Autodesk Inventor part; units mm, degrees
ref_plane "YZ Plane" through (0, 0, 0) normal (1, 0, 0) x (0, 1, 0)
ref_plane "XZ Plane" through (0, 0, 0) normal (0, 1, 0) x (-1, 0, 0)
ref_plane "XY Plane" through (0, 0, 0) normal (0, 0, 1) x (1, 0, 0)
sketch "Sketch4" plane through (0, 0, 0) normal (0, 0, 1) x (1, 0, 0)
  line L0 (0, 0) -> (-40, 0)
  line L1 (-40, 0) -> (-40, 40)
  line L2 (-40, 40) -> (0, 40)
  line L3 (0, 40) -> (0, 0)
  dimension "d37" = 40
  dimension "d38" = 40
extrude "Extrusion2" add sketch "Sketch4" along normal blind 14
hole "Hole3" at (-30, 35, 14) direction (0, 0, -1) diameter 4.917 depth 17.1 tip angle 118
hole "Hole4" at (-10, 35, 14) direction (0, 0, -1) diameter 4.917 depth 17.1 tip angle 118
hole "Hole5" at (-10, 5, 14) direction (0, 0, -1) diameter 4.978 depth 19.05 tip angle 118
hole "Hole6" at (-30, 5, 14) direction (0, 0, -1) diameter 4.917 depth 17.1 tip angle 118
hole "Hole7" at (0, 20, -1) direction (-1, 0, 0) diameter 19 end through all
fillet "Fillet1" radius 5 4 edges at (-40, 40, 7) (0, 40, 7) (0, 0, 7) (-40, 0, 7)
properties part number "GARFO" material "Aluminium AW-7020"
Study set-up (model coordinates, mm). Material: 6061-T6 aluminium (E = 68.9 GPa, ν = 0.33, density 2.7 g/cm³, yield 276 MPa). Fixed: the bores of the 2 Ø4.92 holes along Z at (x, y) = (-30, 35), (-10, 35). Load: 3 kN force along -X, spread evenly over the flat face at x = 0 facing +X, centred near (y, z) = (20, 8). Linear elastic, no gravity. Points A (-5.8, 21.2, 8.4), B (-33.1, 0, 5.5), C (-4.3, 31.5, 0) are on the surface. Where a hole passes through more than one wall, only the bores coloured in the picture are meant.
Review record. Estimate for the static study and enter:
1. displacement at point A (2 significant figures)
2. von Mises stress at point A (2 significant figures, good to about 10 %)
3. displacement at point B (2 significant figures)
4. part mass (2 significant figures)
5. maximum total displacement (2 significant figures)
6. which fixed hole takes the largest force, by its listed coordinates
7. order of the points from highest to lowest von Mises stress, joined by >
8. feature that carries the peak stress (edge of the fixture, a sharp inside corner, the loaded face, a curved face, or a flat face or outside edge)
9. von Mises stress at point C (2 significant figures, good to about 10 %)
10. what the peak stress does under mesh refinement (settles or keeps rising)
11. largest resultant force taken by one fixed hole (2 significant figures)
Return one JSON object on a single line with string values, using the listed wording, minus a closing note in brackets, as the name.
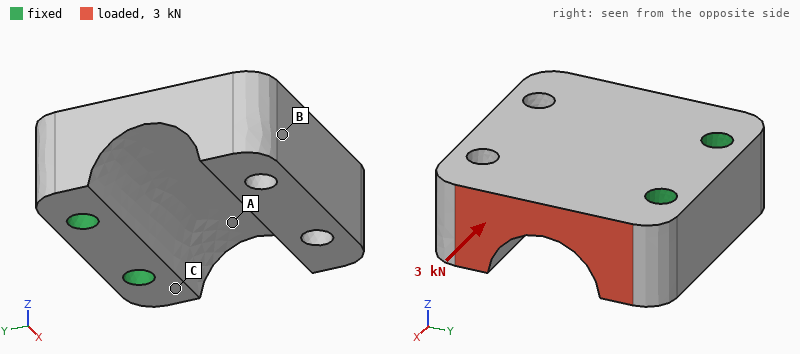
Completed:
{"displacement at point A": "9.0 µm", "von Mises stress at point A": "22 MPa", "displacement at point B": "18 µm", "part mass": "44 g", "maximum total displacement": "22 µm", "which fixed hole takes the largest force, by its listed coordinates": "(-10, 35)", "order of the points from highest to lowest von Mises stress, joined by >": "A > C > B", "feature that carries the peak stress": "edge of the fixture", "von Mises stress at point C": "12 MPa", "what the peak stress does under mesh refinement": "keeps rising", "largest resultant force taken by one fixed hole": "2.6 kN"}
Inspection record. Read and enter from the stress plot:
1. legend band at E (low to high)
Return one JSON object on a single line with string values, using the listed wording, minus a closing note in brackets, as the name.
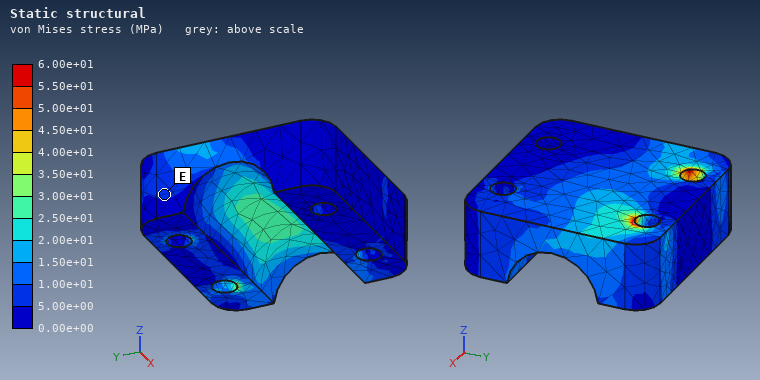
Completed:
{"legend band at E": "5.00e+00 to 1.00e+01 MPa"}
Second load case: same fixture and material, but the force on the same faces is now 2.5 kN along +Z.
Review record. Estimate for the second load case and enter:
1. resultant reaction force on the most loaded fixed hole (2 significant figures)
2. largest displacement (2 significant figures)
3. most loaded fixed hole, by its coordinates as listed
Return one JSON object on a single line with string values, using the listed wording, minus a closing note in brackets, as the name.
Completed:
{"resultant reaction force on the most loaded fixed hole": "2.8 kN", "largest displacement": "0.15 mm", "most loaded fixed hole, by its coordinates as listed": "(-10, 35)"}
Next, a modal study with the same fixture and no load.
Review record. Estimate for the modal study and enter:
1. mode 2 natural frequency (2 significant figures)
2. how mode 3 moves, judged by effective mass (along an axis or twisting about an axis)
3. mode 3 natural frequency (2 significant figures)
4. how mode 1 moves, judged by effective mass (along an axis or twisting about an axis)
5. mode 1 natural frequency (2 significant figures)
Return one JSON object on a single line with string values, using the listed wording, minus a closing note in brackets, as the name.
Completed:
{"mode 2 natural frequency": "8900 Hz", "how mode 3 moves, judged by effective mass": "along X", "mode 3 natural frequency": "12 kHz", "how mode 1 moves, judged by effective mass": "along Z", "mode 1 natural frequency": "4100 Hz"}
